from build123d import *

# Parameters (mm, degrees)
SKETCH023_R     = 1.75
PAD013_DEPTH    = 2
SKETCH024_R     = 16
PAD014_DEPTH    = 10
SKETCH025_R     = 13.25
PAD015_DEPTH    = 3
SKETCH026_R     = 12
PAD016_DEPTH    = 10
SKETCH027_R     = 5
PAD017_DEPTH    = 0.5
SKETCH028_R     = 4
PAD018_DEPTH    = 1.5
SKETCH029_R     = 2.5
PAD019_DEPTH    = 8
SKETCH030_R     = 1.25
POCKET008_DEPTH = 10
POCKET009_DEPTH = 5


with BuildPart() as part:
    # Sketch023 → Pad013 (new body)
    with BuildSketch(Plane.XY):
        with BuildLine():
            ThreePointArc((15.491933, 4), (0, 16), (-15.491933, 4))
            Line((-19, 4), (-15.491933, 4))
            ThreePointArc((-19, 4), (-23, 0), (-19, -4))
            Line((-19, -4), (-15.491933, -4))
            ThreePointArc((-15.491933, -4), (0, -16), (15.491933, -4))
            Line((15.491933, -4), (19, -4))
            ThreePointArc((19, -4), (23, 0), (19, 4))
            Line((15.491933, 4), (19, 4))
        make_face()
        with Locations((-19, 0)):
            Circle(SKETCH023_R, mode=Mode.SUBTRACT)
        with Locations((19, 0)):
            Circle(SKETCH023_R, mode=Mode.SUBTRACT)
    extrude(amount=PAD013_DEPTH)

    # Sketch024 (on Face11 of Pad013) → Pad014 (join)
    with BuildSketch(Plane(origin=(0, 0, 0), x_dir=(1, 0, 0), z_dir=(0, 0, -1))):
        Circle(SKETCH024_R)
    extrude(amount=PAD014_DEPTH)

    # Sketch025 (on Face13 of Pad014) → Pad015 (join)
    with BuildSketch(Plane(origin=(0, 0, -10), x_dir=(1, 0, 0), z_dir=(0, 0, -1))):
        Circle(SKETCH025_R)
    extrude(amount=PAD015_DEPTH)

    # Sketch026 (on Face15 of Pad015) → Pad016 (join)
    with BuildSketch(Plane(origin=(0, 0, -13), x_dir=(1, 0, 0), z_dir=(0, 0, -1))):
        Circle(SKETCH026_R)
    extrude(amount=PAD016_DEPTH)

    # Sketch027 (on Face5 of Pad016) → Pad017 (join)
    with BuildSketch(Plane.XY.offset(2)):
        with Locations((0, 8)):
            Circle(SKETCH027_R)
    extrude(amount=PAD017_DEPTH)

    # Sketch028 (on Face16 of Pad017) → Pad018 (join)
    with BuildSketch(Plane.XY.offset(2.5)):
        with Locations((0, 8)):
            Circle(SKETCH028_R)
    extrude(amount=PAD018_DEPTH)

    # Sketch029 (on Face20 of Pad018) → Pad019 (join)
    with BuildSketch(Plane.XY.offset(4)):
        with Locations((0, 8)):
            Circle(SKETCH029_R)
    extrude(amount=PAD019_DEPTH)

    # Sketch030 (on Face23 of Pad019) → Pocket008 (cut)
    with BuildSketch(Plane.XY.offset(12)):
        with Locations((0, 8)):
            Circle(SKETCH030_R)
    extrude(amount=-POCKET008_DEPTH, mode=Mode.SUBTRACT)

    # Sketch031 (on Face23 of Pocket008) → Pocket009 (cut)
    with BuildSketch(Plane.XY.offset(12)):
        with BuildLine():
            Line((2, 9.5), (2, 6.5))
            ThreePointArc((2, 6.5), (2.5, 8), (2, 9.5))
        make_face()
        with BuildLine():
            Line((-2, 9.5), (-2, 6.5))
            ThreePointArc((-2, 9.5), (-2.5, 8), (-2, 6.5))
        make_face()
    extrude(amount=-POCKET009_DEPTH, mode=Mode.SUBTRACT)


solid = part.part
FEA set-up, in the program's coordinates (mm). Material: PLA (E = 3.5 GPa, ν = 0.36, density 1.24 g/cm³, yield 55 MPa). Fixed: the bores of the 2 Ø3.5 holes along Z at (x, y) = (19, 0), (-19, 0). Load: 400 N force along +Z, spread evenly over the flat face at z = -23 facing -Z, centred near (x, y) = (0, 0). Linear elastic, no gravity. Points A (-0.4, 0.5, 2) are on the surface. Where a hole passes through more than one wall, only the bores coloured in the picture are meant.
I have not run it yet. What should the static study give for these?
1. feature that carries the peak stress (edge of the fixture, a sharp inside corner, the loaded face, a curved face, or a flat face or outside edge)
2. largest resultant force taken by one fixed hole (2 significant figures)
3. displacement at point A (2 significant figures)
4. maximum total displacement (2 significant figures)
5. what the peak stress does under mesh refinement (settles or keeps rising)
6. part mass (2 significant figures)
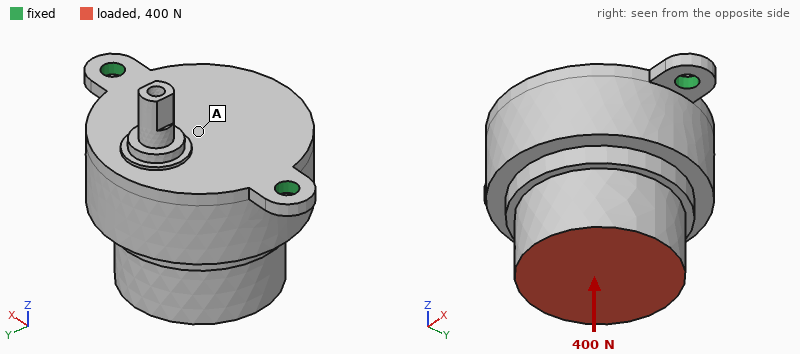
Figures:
edge of the fixture
230 N
67 µm
72 µm
keeps rising
20 g
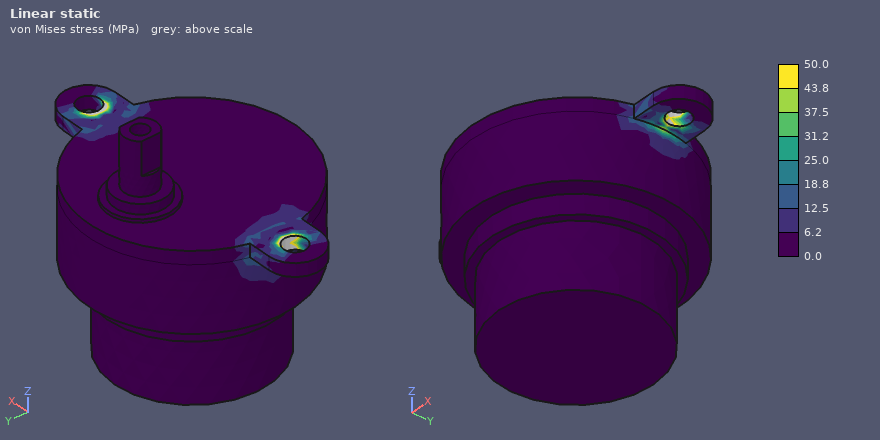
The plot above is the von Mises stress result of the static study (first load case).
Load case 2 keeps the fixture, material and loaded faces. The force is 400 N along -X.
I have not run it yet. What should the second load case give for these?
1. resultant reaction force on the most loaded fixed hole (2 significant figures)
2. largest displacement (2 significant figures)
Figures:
350 N
0.17 mm
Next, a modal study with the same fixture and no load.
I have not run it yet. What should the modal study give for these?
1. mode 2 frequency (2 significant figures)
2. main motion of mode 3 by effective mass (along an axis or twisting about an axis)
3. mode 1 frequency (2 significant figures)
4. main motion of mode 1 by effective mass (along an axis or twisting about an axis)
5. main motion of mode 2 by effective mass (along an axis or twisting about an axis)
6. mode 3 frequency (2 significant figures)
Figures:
2800 Hz
along X
440 Hz
along Y
along Z
3200 Hz
